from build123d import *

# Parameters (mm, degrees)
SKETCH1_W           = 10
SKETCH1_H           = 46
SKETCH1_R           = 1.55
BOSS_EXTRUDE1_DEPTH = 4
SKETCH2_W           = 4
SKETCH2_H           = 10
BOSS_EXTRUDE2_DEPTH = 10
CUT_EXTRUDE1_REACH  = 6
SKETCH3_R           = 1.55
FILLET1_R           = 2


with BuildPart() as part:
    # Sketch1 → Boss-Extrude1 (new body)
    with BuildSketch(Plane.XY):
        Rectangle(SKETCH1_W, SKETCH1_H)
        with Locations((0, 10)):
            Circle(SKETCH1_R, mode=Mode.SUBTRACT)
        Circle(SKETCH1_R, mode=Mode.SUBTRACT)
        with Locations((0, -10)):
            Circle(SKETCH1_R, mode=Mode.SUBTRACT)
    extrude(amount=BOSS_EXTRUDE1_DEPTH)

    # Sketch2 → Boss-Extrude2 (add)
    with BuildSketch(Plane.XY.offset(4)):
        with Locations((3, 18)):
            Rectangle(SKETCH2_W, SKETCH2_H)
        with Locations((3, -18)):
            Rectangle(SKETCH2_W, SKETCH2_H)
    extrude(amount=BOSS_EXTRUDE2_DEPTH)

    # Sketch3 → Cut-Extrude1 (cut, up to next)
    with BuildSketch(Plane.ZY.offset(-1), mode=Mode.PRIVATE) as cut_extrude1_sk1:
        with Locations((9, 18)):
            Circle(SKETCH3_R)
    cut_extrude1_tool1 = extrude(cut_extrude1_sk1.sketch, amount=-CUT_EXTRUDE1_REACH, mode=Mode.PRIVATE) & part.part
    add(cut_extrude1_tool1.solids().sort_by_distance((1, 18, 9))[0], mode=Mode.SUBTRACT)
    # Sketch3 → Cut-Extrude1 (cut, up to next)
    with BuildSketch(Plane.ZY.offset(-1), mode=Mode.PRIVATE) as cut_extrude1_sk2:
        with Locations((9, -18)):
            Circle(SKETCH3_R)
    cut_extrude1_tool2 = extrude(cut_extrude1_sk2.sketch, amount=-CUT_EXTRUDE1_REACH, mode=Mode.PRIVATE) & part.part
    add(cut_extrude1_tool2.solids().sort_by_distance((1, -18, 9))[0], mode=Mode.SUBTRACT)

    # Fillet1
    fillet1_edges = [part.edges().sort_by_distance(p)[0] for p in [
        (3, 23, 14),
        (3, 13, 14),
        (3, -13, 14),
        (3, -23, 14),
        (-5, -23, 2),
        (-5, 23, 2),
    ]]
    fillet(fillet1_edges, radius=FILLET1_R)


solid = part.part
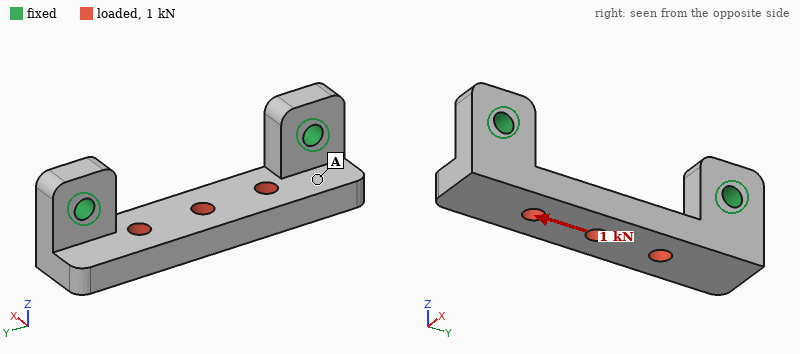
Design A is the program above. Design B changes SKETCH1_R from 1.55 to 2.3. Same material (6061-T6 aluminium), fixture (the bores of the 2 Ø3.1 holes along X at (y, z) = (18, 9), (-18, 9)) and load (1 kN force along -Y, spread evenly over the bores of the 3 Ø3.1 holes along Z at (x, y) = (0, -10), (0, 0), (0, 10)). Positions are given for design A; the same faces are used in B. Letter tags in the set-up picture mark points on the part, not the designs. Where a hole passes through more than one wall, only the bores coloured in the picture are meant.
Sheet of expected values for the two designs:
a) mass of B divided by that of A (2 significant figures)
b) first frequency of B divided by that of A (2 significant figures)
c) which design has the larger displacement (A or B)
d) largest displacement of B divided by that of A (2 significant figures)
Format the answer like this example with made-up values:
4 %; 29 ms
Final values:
0.96; 1.0; B; 1.1
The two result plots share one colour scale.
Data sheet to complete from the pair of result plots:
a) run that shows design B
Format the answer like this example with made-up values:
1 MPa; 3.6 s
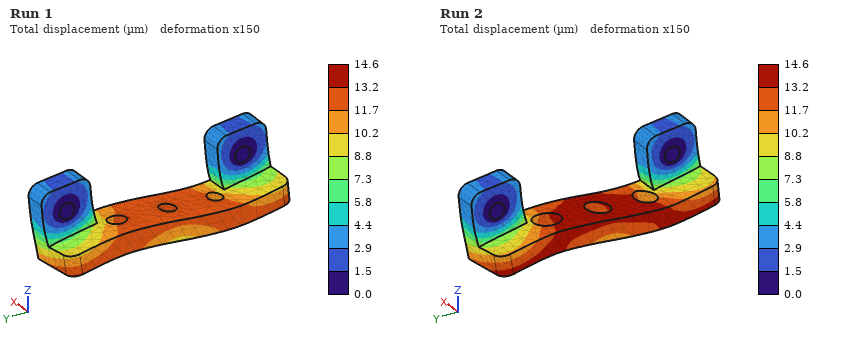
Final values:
Run 2
